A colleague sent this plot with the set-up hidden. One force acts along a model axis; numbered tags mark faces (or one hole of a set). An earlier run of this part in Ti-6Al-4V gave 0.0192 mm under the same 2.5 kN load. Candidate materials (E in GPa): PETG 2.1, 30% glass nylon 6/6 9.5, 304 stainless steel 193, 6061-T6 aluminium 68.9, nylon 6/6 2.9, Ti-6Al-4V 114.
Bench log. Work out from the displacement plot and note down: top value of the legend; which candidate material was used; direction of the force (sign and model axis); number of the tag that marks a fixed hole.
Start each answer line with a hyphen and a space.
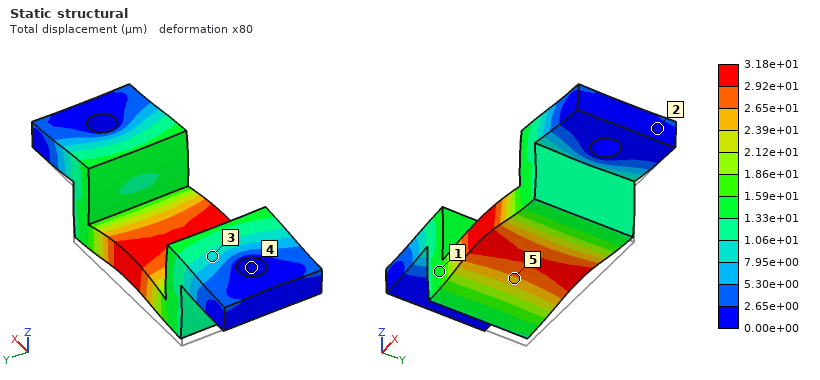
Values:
- 3.18e+01 µm
- 6061-T6 aluminium
- +Z
- 4
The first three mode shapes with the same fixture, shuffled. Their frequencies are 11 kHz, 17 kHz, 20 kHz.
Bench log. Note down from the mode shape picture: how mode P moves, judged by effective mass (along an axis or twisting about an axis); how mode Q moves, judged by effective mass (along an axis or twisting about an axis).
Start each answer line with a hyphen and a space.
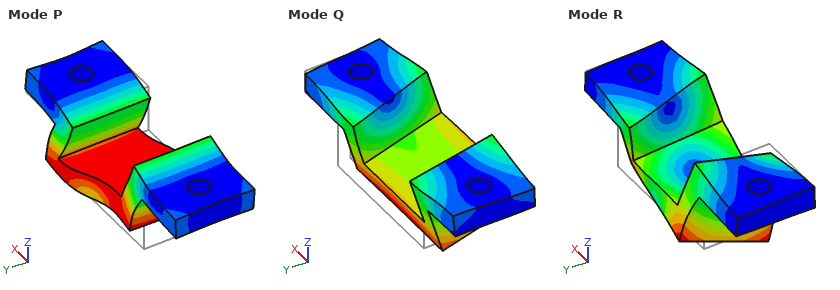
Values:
- along X
- along Y
